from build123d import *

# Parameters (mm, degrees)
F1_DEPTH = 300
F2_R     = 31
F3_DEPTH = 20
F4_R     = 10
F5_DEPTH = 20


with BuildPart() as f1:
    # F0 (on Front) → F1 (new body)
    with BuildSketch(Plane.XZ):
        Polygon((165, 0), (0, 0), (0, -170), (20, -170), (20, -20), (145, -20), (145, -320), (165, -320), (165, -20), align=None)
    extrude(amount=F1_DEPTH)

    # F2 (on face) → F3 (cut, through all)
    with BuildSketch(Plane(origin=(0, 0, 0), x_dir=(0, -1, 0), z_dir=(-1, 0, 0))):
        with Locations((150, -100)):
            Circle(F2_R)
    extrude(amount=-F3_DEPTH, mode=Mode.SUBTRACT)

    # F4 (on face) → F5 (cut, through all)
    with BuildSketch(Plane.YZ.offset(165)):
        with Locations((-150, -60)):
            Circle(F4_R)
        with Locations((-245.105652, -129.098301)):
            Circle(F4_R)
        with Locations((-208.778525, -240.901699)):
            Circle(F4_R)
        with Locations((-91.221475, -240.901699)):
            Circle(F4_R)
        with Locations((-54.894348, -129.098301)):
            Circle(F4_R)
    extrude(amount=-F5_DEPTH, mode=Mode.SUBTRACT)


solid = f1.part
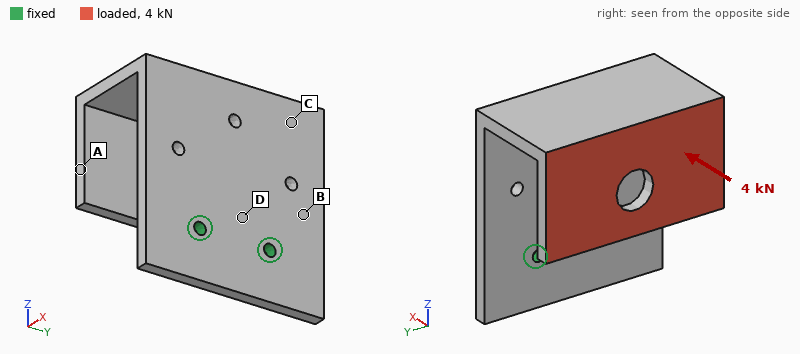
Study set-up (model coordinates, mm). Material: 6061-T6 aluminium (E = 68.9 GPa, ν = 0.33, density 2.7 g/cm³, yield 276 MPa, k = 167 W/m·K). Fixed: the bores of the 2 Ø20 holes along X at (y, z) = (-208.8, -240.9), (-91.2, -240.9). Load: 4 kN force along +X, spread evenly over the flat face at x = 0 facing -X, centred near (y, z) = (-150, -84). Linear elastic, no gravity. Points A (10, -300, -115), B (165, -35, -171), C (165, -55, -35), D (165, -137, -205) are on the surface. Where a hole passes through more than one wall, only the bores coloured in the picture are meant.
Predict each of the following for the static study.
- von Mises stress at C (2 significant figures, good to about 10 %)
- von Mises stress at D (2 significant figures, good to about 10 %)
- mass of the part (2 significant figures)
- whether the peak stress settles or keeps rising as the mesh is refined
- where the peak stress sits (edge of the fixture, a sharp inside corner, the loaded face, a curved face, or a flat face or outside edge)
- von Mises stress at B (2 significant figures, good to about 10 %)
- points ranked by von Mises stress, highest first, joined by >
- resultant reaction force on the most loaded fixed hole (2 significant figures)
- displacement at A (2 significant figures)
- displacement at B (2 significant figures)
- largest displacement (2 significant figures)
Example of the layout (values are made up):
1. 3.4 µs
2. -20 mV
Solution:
1. 8.5 MPa
2. 23 MPa
3. 9.7 kg
4. keeps rising
5. edge of the fixture
6. 15 MPa
7. D > B > C > A
8. 2.0 kN
9. 0.75 mm
10. 0.12 mm
11. 0.78 mm
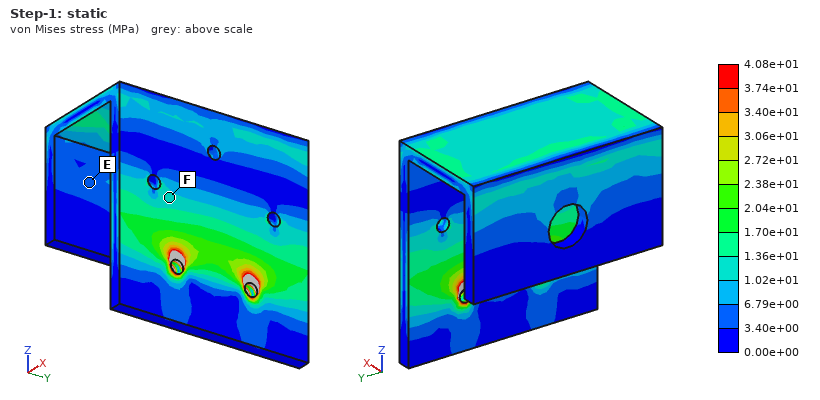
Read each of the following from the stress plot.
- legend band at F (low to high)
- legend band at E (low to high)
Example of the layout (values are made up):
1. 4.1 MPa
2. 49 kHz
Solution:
1. 1.02e+01 to 1.36e+01 MPa
2. 3.40e+00 to 6.79e+00 MPa
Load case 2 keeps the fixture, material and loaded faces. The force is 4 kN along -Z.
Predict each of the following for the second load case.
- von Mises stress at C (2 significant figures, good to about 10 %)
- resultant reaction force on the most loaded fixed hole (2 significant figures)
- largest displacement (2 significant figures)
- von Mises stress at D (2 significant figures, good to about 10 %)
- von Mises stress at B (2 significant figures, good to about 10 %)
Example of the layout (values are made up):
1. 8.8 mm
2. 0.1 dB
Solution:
1. 27 MPa
2. 2.0 kN
3. 2.3 mm
4. 29 MPa
5. 28 MPa
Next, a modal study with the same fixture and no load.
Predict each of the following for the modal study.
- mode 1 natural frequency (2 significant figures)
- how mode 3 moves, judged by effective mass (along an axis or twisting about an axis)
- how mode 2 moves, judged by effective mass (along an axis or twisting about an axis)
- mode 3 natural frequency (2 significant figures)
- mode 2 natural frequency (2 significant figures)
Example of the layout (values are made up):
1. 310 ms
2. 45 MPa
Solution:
1. 100 Hz
2. along X
3. along Y
4. 210 Hz
5. 160 Hz
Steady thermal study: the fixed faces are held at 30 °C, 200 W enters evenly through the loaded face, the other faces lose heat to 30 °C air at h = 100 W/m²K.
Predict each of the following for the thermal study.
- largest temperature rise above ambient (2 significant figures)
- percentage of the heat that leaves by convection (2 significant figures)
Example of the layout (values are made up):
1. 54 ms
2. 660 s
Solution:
1. 19 K
2. 96 %
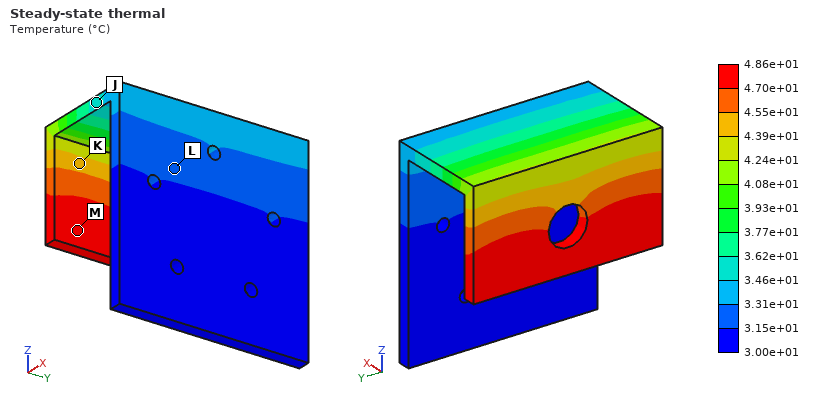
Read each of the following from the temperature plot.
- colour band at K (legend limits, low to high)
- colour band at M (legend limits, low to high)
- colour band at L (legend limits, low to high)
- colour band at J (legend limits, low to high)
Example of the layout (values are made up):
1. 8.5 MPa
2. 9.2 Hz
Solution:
1. 4.39e+01 to 4.55e+01 °C
2. 4.70e+01 to 4.86e+01 °C
3. 3.15e+01 to 3.31e+01 °C
4. 3.46e+01 to 3.62e+01 °C
